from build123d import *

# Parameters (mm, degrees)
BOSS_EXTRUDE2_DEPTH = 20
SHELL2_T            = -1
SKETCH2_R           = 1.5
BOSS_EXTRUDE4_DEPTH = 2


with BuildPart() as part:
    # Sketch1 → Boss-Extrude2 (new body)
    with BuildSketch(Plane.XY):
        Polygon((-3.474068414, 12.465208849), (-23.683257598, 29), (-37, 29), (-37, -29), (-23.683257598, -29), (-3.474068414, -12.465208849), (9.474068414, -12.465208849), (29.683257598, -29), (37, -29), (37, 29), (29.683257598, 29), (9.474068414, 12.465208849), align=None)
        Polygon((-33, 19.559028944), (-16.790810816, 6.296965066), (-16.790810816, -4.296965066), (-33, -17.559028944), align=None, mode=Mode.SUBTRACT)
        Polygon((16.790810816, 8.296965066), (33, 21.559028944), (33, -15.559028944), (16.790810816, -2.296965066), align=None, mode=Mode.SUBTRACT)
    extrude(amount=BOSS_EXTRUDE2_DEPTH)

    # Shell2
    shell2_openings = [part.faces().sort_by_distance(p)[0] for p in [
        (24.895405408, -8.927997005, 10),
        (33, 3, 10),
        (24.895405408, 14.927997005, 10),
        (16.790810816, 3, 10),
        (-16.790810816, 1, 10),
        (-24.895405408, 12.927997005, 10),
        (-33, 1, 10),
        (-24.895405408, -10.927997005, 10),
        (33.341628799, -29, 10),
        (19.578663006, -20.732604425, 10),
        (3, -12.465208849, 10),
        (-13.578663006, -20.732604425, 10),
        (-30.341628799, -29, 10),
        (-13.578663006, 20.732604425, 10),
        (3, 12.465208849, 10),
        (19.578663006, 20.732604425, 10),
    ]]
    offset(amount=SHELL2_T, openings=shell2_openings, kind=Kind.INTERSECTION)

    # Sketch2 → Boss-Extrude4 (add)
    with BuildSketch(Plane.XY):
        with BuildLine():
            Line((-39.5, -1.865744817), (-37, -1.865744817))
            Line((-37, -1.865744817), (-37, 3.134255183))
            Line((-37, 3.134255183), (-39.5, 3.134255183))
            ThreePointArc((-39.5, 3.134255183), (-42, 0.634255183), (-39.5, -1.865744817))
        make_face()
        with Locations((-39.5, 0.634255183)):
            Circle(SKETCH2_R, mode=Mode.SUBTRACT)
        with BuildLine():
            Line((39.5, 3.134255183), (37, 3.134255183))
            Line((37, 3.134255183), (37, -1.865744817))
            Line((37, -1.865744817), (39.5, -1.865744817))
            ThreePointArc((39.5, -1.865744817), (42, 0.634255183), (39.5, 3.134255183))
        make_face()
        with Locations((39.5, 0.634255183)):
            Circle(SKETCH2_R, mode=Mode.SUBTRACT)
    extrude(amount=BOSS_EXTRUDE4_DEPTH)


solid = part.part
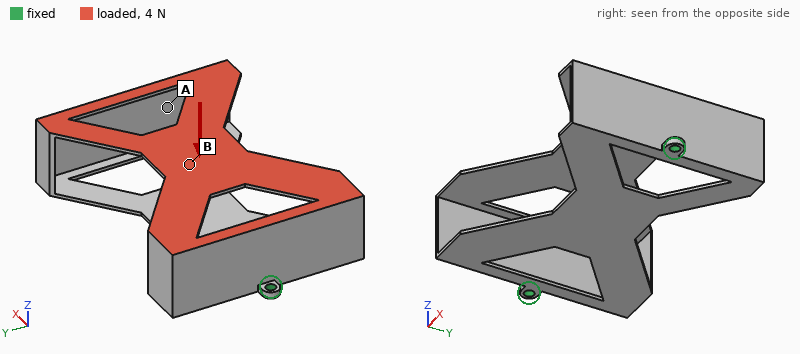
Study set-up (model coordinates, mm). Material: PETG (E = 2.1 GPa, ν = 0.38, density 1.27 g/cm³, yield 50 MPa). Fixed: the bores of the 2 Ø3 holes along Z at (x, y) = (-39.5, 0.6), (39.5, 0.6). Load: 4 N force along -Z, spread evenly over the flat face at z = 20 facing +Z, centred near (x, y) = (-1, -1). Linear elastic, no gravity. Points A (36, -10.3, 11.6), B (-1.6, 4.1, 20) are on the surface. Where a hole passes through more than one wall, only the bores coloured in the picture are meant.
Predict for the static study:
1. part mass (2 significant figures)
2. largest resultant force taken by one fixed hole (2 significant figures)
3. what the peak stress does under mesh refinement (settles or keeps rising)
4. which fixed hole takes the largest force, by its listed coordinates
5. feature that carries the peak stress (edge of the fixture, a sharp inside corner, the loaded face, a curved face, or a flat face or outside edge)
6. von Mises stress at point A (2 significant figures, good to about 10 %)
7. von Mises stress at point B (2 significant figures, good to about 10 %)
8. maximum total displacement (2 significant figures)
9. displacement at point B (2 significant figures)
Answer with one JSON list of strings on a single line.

["9.3 g", "2.1 N", "keeps rising", "(-39.5, 0.6)", "a sharp inside corner", "0.77 MPa", "2.1 MPa", "1.1 mm", "0.92 mm"]
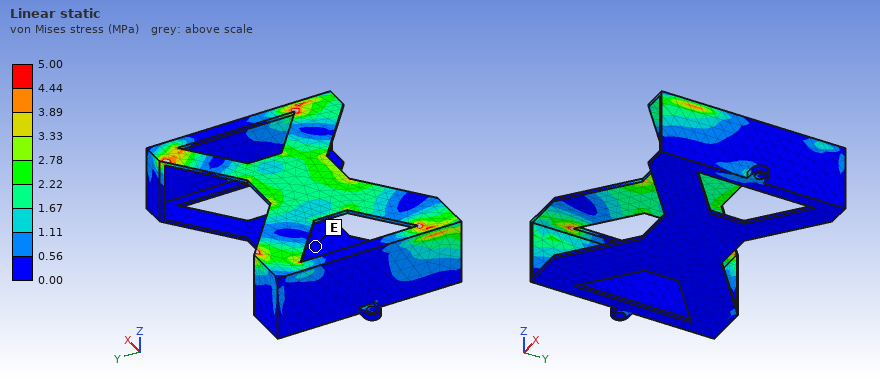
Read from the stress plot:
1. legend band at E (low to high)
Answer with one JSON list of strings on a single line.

["0.00 to 0.56 MPa"]
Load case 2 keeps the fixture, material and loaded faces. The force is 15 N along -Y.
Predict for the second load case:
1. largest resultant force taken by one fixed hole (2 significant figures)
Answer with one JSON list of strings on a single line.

["7.8 N"]
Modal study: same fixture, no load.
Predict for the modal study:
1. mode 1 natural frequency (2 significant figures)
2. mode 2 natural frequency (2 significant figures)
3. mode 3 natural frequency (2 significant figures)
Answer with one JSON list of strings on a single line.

["200 Hz", "200 Hz", "220 Hz"]
